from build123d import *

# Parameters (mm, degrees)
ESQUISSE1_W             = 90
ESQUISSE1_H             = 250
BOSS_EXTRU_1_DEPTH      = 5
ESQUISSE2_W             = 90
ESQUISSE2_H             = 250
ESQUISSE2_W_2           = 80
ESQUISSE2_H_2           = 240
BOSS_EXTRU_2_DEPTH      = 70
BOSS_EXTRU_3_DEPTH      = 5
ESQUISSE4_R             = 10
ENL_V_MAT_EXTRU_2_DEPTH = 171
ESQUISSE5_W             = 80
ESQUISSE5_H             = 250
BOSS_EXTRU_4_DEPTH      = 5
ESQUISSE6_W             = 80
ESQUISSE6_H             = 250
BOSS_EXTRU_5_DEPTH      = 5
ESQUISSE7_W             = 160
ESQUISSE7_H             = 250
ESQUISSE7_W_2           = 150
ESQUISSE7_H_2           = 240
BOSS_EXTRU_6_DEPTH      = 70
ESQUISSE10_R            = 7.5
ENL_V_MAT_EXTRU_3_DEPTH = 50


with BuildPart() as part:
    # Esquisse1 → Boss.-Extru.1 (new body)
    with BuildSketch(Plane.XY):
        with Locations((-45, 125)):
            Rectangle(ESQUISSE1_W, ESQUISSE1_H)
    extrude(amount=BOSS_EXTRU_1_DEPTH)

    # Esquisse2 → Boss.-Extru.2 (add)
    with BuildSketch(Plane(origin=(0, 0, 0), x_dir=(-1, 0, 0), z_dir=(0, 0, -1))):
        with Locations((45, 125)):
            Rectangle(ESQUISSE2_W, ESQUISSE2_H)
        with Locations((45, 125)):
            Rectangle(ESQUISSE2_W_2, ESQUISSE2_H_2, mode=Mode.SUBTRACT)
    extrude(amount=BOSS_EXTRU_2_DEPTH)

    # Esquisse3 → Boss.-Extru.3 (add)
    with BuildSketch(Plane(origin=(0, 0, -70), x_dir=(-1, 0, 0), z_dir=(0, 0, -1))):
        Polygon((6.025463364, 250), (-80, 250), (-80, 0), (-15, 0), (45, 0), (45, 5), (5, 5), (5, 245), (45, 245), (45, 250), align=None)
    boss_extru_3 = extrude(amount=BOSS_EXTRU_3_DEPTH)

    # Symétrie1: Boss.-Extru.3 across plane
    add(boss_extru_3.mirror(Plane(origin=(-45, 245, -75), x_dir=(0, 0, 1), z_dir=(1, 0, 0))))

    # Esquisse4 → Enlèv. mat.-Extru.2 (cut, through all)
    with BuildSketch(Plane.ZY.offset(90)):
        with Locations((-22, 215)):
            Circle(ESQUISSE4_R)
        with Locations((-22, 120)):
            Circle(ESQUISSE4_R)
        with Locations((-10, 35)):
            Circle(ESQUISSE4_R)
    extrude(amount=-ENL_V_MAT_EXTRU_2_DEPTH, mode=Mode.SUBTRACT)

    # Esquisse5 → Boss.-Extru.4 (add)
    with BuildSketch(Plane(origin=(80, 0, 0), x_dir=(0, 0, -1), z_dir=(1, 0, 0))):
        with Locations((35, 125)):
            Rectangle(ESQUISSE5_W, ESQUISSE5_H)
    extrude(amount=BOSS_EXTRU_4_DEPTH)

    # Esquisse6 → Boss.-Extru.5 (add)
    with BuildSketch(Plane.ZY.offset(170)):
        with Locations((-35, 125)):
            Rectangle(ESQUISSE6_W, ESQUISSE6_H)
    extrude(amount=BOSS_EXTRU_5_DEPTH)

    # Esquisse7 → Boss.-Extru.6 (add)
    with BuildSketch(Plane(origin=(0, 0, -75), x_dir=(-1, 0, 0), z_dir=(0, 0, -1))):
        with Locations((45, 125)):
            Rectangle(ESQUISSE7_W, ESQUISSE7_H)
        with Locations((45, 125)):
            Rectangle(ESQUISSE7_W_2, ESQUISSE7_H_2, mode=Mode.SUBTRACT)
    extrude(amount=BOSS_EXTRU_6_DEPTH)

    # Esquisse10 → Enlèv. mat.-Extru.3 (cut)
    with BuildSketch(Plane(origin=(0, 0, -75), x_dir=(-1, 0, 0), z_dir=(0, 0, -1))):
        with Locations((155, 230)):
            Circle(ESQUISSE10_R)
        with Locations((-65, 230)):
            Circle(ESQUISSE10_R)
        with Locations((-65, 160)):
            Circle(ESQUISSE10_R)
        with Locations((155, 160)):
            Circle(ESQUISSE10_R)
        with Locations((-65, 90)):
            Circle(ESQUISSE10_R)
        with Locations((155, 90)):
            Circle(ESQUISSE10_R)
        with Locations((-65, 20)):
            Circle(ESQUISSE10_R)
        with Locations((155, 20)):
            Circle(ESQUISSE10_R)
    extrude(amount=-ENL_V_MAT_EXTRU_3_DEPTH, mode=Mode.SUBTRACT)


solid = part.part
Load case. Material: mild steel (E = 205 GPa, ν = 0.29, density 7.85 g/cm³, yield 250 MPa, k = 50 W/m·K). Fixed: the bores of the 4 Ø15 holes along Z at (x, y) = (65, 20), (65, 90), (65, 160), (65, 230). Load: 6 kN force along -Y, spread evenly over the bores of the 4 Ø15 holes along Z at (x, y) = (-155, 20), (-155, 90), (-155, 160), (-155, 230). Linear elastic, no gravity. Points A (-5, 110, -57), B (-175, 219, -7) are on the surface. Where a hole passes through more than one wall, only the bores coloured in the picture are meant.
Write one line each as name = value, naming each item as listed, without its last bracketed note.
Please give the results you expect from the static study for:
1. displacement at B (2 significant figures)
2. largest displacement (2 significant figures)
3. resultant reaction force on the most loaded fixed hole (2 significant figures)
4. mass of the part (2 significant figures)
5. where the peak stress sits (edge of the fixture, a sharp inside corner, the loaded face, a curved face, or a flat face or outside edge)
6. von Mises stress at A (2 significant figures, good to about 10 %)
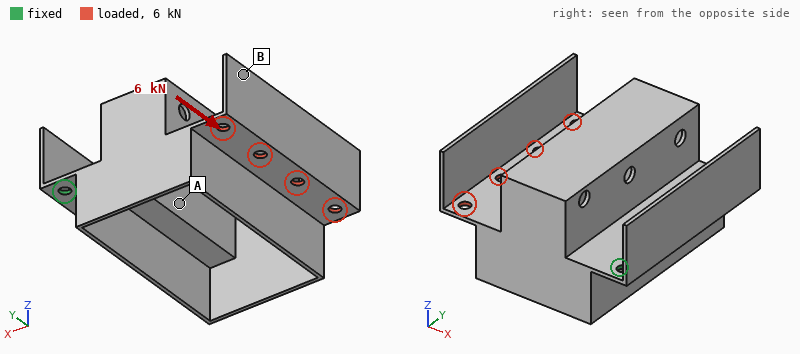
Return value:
displacement at B = 0.93 mm
largest displacement = 1.7 mm
resultant reaction force on the most loaded fixed hole = 6.1 kN
mass of the part = 8.0 kg
where the peak stress sits = a flat face or outside edge
von Mises stress at A = 37 MPa
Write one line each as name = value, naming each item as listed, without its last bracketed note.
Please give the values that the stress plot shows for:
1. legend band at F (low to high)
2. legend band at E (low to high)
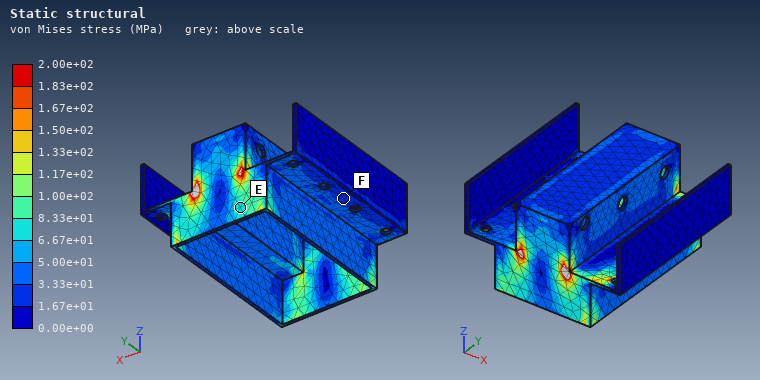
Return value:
legend band at F = 1.67e+01 to 3.33e+01 MPa
legend band at E = 6.67e+01 to 8.33e+01 MPa
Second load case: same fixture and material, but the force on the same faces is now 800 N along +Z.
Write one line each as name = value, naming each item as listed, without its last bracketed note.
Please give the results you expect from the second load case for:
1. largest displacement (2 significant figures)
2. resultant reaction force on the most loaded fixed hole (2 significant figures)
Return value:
largest displacement = 2.4 mm
resultant reaction force on the most loaded fixed hole = 870 N
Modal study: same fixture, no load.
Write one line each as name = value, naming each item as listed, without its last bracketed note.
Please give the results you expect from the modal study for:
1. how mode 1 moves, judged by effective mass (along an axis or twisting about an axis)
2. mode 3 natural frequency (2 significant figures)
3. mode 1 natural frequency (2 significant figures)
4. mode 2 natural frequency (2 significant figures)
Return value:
how mode 1 moves, judged by effective mass = along Z
mode 3 natural frequency = 320 Hz
mode 1 natural frequency = 56 Hz
mode 2 natural frequency = 170 Hz
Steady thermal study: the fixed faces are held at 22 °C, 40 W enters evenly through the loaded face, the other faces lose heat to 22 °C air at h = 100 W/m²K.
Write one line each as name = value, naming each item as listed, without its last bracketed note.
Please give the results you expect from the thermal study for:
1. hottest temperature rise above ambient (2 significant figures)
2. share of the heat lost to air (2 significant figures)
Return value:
hottest temperature rise above ambient = 15 K
share of the heat lost to air = 100 %
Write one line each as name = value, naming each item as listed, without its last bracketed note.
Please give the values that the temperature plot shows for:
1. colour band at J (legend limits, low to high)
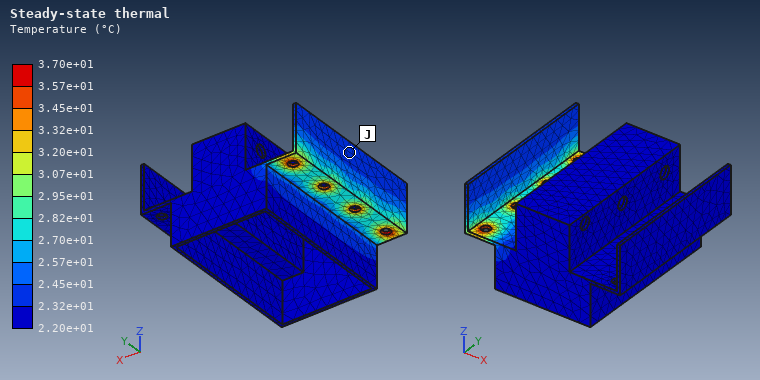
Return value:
colour band at J = 2.32e+01 to 2.45e+01 °C
